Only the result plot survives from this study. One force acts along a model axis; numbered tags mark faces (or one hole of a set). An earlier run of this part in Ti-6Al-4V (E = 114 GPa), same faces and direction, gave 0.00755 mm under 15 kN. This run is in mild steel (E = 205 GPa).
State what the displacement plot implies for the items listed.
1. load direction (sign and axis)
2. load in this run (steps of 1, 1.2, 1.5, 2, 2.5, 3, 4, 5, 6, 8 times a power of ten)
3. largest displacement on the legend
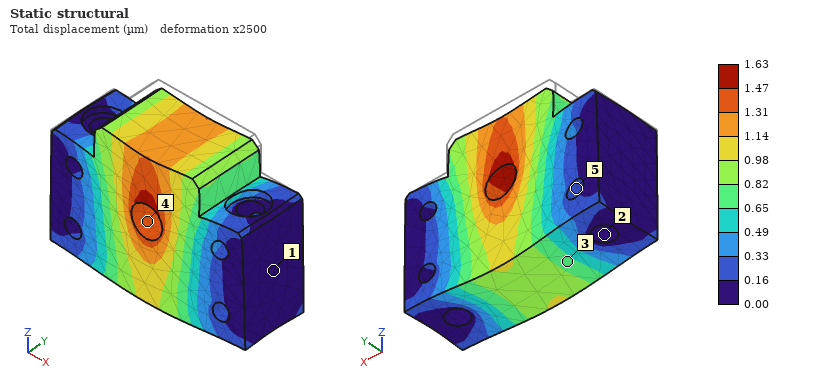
-Z
6 kN
1.63 µm
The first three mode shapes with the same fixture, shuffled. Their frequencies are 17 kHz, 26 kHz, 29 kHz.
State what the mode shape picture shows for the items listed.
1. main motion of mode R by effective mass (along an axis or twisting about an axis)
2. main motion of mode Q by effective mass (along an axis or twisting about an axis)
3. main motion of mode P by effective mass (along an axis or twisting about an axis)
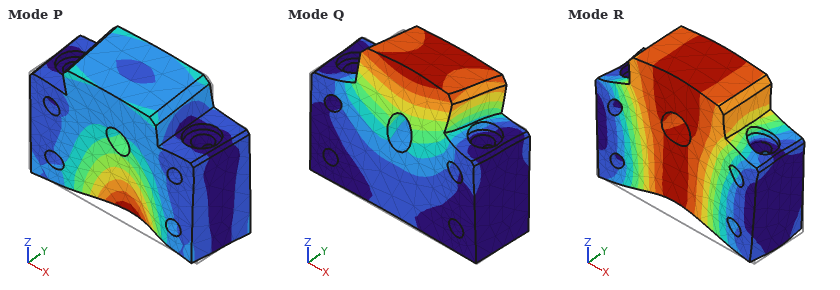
along Z
along Y
along Y
